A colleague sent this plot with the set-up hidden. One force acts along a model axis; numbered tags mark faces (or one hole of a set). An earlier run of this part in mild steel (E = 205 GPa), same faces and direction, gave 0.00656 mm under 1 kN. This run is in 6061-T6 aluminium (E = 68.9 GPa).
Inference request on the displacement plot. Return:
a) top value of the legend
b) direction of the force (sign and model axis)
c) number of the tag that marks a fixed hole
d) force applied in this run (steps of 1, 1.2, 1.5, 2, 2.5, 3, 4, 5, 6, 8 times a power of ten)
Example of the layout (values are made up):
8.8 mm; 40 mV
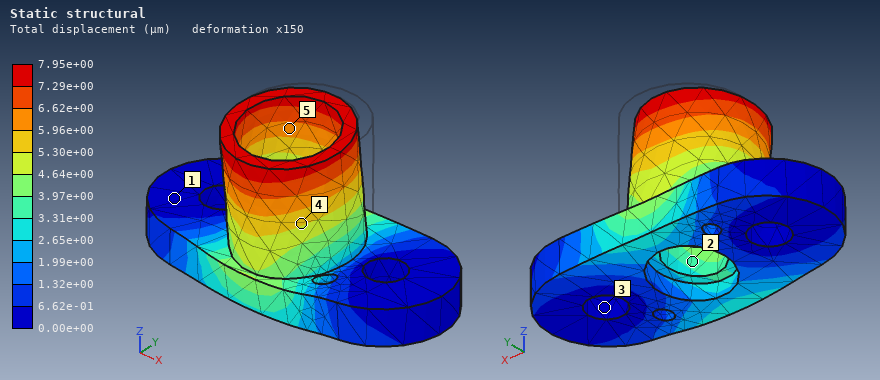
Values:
7.95e+00 µm; -Y; 3; 400 N
